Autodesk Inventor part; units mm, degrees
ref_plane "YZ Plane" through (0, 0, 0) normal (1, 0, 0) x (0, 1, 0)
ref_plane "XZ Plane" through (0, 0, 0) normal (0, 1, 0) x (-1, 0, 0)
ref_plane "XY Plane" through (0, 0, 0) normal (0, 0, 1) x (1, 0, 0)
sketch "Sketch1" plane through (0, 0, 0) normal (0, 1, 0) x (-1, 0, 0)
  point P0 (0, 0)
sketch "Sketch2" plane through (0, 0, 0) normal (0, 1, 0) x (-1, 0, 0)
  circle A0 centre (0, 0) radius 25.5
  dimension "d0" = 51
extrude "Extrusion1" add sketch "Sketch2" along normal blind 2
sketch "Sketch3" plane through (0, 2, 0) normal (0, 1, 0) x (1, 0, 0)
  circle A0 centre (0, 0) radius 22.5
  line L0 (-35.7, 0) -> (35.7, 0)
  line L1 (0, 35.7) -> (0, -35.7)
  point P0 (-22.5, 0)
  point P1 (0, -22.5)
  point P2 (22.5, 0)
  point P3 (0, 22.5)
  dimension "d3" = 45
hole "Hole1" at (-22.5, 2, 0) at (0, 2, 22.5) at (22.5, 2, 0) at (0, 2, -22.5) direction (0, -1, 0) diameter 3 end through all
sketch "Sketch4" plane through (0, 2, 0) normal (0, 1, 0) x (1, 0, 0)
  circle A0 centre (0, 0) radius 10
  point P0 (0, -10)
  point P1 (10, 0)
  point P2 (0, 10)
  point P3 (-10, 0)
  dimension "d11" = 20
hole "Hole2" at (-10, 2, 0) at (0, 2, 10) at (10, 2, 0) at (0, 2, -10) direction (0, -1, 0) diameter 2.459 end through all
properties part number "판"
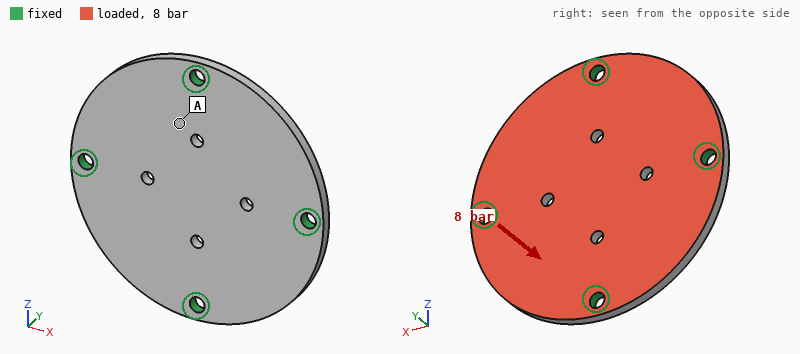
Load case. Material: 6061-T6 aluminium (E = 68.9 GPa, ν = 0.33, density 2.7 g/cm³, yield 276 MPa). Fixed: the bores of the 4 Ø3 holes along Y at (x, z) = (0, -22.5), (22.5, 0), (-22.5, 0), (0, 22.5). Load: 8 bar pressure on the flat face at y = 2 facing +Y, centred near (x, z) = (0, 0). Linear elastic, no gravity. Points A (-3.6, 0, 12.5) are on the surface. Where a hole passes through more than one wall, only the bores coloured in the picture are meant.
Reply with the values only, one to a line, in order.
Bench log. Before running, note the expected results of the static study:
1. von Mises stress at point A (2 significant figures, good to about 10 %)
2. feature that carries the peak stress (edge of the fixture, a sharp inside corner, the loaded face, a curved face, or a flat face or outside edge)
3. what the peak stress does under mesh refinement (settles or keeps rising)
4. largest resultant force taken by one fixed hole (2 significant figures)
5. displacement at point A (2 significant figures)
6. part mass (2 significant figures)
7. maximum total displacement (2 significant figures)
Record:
39 MPa
edge of the fixture
keeps rising
400 N
56 µm
11 g
95 µm
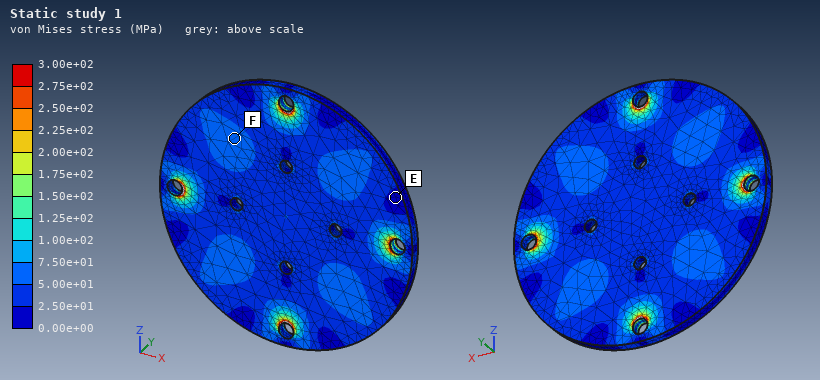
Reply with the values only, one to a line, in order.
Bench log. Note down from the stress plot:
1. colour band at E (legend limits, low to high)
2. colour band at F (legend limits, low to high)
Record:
0.00e+00 to 2.50e+01 MPa
5.00e+01 to 7.50e+01 MPa
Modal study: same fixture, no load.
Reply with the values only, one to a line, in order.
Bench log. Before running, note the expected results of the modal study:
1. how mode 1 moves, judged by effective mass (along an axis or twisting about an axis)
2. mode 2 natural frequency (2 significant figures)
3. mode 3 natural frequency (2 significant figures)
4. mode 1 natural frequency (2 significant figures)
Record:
along Y
9000 Hz
9400 Hz
7600 Hz
